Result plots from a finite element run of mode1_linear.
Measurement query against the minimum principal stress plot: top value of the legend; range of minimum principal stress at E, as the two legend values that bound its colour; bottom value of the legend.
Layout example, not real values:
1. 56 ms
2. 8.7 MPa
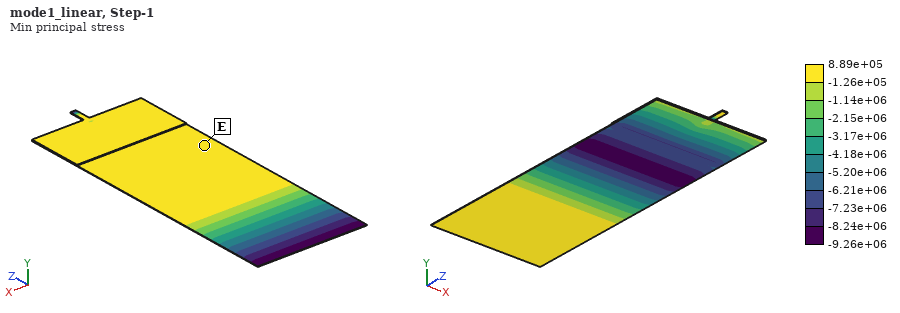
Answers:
1. 8.89e+05
2. -1.26e+05 to 8.89e+05
3. -9.26e+06
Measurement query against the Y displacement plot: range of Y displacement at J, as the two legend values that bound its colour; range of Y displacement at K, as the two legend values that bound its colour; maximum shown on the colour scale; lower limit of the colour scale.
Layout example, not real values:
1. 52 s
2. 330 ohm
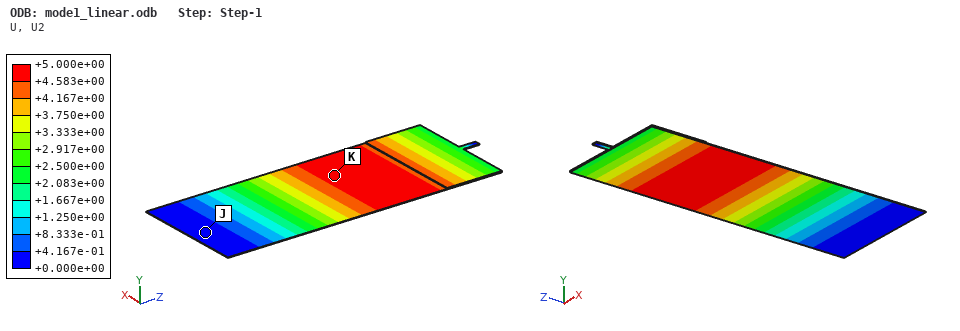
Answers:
1. +0.000e+00 to +4.167e-01
2. +4.583e+00 to +5.000e+00
3. +5.000e+00
4. +0.000e+00
